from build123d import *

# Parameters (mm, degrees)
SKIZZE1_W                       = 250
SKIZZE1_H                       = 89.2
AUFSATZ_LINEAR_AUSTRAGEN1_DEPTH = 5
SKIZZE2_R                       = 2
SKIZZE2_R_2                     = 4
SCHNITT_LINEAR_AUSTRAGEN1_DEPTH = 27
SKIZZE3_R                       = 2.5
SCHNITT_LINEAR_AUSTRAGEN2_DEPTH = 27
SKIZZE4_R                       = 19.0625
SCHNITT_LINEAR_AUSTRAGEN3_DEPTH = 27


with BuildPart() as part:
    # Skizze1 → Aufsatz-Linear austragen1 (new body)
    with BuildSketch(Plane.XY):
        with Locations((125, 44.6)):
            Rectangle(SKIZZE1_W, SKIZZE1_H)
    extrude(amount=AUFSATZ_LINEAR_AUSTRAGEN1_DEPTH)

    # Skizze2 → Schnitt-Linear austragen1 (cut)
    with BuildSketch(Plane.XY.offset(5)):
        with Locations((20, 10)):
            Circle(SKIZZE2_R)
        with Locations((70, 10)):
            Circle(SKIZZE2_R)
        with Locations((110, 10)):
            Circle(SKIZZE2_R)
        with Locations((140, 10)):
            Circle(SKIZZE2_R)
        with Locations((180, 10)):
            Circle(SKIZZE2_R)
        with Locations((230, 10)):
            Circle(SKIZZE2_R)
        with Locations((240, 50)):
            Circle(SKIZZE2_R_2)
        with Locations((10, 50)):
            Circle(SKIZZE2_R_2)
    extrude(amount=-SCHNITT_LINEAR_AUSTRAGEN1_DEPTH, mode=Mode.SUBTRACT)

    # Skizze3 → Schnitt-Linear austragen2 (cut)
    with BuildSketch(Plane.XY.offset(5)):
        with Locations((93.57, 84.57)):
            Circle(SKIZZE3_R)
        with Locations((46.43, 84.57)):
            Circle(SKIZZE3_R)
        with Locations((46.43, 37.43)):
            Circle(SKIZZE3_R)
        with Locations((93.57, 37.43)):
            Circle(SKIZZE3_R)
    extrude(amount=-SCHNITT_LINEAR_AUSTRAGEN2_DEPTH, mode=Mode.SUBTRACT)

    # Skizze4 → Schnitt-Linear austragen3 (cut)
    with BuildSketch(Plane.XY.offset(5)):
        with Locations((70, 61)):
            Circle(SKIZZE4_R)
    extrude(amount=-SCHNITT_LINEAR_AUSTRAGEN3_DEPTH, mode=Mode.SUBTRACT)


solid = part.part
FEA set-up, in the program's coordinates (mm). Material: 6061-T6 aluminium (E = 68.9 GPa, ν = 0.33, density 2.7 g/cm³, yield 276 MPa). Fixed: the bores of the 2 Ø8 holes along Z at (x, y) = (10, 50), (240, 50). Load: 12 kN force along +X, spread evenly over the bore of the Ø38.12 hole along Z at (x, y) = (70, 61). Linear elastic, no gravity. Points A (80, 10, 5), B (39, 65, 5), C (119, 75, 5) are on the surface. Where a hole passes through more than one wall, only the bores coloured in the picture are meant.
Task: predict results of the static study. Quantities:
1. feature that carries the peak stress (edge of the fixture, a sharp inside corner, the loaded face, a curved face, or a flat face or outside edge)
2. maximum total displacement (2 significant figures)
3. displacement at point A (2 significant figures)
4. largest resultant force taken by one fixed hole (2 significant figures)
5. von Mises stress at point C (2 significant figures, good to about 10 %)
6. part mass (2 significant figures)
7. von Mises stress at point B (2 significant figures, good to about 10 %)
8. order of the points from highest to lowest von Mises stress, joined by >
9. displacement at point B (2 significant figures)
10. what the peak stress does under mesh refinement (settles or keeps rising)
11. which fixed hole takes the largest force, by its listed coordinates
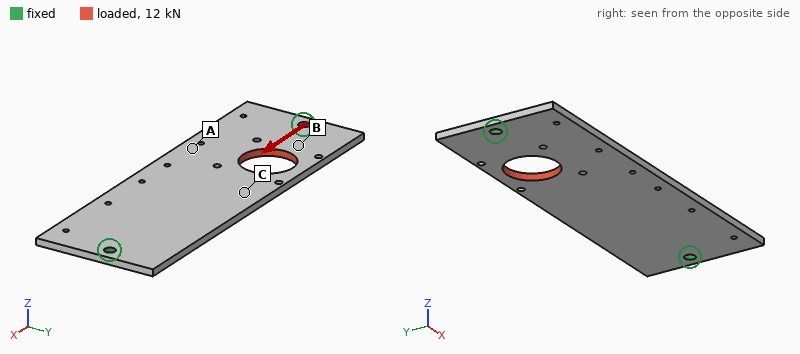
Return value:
edge of the fixture
51 µm
21 µm
7.6 kN
20 MPa
280 g
33 MPa
B > C > A
27 µm
keeps rising
(10, 50)
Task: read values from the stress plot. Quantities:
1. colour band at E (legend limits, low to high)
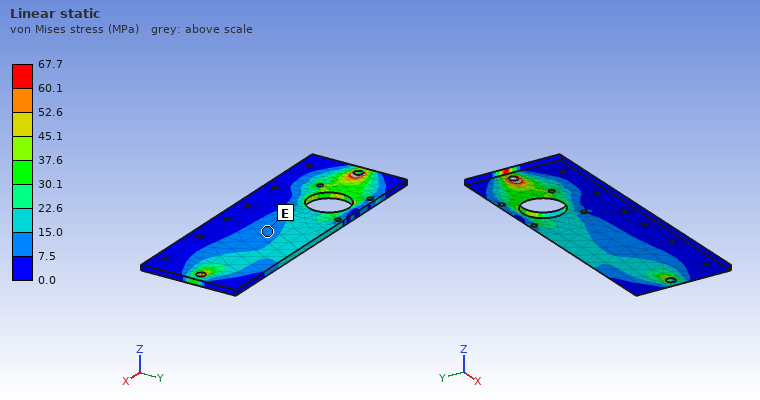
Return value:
7.5 to 15.0 MPa
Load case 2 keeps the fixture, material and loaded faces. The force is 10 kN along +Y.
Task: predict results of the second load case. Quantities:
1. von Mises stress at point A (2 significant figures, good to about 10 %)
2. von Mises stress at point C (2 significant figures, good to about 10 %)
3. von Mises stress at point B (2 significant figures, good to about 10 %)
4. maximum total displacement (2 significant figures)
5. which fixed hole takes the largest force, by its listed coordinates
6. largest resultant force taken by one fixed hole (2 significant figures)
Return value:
45 MPa
22 MPa
44 MPa
0.15 mm
(10, 50)
7.6 kN
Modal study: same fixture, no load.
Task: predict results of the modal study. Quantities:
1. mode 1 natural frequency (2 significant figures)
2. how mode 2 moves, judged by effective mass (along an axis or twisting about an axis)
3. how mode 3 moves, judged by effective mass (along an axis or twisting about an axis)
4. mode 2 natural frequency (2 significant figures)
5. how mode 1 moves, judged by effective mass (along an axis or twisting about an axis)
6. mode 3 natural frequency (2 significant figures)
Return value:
440 Hz
twisting about X
twisting about Y
660 Hz
along Z
1100 Hz
